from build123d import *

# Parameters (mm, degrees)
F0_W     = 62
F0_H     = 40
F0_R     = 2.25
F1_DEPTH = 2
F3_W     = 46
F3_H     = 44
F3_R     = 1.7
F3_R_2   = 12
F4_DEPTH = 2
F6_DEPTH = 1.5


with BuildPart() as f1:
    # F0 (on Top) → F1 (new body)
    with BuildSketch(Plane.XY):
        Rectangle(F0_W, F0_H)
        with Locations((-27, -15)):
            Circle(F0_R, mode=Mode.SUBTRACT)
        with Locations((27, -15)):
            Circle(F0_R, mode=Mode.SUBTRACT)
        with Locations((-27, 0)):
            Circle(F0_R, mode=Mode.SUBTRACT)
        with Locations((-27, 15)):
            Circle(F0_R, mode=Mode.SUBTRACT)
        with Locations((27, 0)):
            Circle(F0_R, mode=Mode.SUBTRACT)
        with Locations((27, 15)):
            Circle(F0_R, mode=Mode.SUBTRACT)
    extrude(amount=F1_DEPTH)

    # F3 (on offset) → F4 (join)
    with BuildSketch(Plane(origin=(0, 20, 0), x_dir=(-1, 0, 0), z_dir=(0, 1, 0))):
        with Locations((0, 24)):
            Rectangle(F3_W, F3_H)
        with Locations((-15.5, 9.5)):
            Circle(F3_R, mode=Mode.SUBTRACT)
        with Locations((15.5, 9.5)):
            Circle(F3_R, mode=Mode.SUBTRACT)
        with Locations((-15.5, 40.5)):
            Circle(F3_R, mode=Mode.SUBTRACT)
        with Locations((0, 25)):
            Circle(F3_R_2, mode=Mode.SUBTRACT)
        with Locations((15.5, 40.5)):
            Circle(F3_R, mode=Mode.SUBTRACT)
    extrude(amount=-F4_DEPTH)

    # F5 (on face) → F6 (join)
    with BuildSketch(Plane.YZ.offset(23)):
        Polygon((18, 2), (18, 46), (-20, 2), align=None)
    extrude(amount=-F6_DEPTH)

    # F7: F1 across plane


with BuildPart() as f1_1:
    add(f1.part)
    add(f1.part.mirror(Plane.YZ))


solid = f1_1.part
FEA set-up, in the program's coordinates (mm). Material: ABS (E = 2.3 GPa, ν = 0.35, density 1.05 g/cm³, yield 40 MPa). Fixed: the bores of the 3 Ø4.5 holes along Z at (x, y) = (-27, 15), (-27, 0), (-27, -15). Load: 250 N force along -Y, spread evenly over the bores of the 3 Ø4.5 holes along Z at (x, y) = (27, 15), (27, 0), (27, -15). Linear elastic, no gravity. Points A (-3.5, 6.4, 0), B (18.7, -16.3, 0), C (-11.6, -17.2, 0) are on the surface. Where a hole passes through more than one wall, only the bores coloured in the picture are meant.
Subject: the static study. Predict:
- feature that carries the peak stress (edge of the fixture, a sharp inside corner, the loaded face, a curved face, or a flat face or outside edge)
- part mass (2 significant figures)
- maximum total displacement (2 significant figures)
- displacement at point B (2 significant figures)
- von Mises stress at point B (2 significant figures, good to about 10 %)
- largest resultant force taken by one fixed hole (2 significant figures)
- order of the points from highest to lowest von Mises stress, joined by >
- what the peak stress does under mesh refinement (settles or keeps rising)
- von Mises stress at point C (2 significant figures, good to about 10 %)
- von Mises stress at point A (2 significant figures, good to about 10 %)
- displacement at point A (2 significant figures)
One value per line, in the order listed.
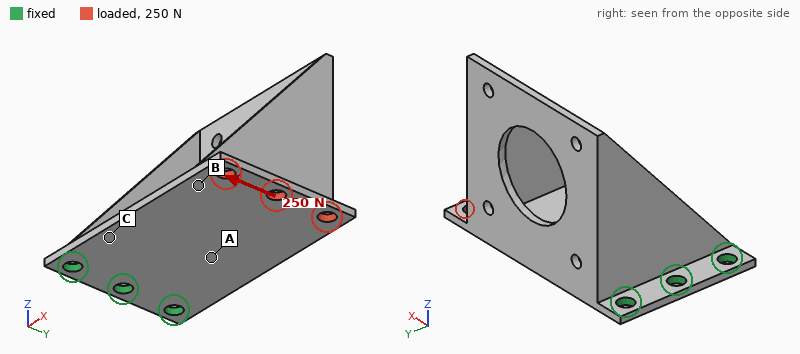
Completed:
edge of the fixture
11 g
0.95 mm
0.67 mm
3.7 MPa
430 N
C > A > B
keeps rising
14 MPa
8.1 MPa
0.23 mm
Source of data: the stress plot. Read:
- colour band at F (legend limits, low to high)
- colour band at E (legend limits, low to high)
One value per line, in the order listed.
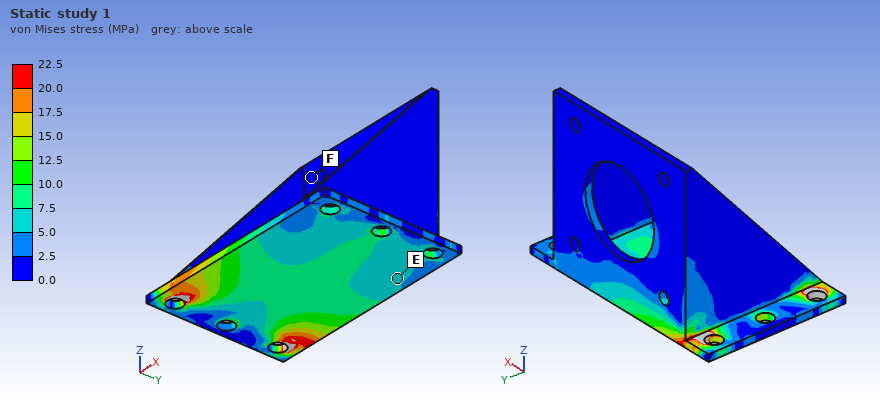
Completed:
0.0 to 2.5 MPa
5.0 to 7.5 MPa
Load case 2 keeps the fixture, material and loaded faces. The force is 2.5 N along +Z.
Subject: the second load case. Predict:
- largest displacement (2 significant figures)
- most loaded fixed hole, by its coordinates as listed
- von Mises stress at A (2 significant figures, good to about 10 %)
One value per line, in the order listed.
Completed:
0.97 mm
(-27, 0)
0.53 MPa
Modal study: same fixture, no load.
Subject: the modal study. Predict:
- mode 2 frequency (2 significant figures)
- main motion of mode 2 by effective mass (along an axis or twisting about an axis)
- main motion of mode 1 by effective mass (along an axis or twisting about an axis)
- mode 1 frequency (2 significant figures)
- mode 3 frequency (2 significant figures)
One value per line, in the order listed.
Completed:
270 Hz
along Y
along Z
130 Hz
920 Hz
